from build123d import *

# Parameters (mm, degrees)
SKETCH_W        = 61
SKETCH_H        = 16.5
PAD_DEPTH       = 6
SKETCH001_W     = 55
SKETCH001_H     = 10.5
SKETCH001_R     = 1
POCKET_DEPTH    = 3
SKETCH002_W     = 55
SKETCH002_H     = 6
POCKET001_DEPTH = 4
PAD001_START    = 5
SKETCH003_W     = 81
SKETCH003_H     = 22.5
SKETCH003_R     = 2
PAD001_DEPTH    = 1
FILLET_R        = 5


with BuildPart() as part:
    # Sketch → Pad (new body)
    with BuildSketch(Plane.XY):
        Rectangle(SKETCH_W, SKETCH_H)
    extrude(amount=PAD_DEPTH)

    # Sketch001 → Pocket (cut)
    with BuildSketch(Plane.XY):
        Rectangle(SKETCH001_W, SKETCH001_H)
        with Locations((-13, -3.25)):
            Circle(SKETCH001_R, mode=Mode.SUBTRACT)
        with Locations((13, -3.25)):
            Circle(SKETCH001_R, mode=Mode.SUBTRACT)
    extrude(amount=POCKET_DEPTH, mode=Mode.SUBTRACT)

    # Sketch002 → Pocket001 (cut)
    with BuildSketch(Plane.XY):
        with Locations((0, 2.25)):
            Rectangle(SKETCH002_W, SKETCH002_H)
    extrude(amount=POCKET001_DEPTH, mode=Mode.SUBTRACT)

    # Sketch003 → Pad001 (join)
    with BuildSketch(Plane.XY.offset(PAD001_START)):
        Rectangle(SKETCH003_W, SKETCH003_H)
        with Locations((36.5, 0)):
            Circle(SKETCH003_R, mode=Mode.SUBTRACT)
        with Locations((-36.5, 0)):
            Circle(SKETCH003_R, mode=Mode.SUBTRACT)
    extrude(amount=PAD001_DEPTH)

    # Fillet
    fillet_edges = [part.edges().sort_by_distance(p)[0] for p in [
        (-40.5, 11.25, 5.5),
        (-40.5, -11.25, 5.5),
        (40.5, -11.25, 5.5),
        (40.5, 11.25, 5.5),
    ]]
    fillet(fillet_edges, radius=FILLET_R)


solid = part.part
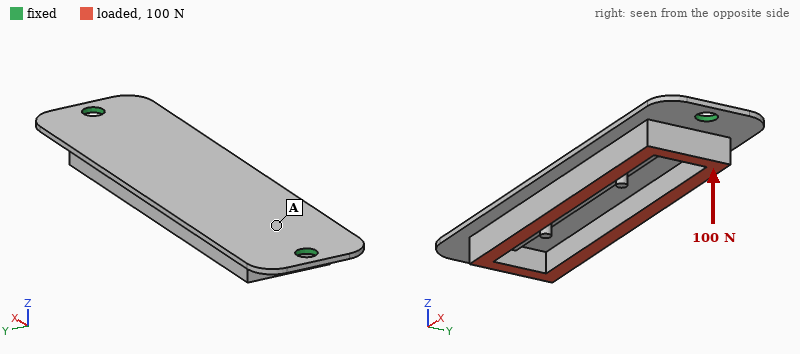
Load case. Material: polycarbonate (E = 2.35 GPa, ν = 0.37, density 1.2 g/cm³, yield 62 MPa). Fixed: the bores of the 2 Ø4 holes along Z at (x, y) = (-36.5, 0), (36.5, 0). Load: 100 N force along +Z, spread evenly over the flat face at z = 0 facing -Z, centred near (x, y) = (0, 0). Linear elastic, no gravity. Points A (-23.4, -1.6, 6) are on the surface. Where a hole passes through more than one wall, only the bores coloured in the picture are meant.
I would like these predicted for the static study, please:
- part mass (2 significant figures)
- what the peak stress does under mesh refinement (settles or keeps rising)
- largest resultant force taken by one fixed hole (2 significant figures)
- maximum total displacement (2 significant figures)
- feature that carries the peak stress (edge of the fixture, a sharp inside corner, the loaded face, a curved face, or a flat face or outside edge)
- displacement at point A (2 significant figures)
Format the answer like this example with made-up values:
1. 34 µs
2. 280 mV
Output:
1. 5.7 g
2. keeps rising
3. 120 N
4. 0.89 mm
5. edge of the fixture
6. 0.51 mm
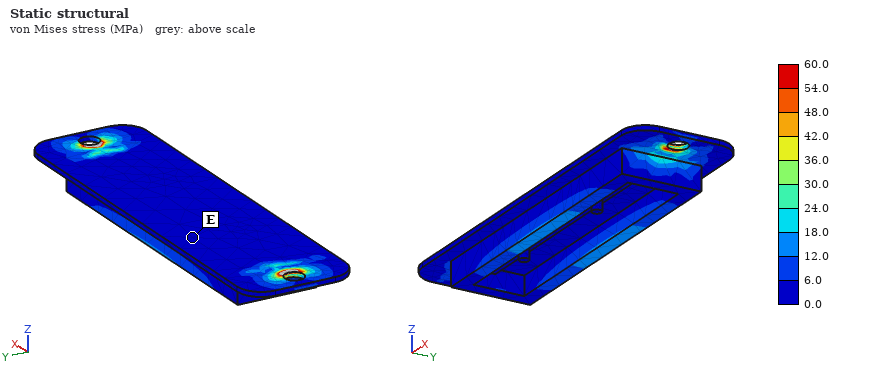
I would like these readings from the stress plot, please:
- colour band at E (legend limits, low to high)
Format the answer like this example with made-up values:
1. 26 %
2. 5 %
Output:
1. 0.0 to 6.0 MPa
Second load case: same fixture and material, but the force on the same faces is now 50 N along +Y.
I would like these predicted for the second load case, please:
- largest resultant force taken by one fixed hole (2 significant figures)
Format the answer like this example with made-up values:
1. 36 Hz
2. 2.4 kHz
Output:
1. 25 N
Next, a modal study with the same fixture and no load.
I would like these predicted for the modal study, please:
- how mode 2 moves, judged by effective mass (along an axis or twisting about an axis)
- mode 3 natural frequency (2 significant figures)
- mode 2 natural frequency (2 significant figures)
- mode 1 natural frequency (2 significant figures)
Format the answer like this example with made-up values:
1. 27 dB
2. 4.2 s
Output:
1. along Z
2. 1900 Hz
3. 810 Hz
4. 650 Hz
